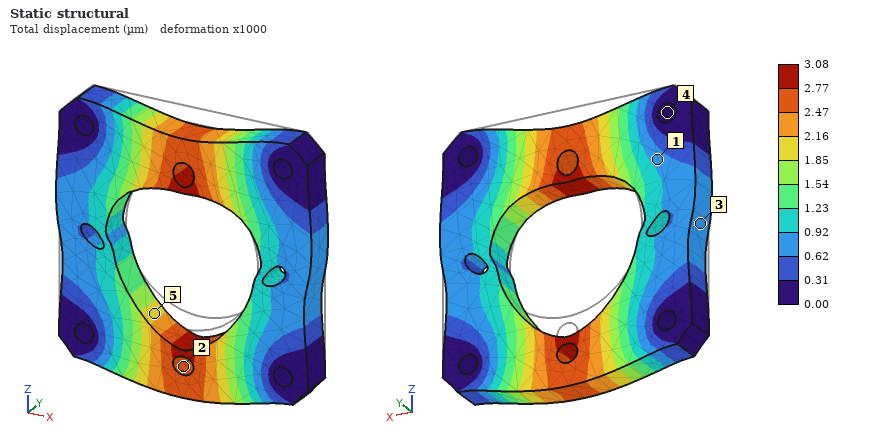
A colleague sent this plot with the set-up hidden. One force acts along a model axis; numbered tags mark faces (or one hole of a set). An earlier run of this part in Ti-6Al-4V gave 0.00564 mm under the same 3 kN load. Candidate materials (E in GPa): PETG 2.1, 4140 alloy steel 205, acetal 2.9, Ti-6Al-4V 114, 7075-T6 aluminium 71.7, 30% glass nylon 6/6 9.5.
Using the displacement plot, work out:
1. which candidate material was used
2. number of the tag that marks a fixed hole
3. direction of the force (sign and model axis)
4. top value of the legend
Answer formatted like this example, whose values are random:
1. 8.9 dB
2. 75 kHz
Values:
1. 4140 alloy steel
2. 4
3. -Z
4. 3.08 µm
